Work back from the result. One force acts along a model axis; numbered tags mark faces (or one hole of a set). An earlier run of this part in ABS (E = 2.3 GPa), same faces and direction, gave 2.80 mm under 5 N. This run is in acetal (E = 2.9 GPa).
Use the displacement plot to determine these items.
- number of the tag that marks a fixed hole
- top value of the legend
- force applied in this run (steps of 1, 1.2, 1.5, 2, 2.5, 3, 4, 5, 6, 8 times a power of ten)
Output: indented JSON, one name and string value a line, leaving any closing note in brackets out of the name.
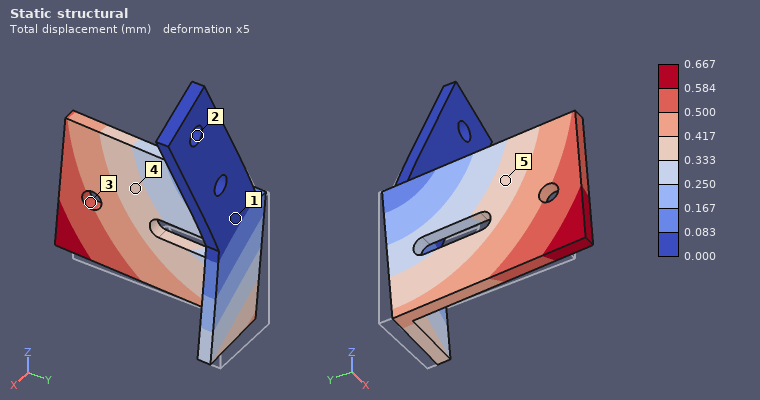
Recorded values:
{
  "number of the tag that marks a fixed hole": "2",
  "top value of the legend": "0.667 mm",
  "force applied in this run": "1.5 N"
}
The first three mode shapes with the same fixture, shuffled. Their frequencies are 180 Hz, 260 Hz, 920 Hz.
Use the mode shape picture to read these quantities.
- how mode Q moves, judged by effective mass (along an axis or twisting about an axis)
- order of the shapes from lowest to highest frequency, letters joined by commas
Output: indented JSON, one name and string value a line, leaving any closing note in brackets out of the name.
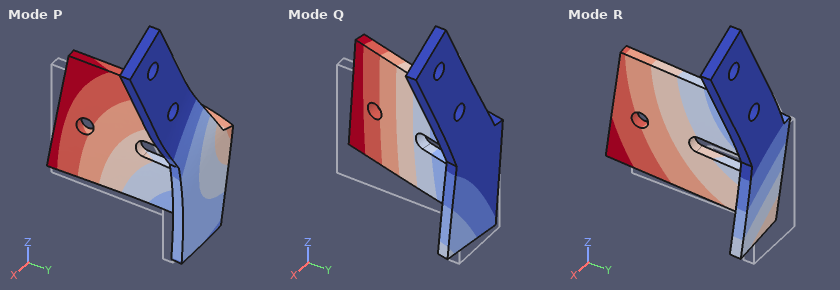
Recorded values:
{
  "how mode Q moves, judged by effective mass": "along X",
  "order of the shapes from lowest to highest frequency, letters joined by commas": "R, Q, P"
}
